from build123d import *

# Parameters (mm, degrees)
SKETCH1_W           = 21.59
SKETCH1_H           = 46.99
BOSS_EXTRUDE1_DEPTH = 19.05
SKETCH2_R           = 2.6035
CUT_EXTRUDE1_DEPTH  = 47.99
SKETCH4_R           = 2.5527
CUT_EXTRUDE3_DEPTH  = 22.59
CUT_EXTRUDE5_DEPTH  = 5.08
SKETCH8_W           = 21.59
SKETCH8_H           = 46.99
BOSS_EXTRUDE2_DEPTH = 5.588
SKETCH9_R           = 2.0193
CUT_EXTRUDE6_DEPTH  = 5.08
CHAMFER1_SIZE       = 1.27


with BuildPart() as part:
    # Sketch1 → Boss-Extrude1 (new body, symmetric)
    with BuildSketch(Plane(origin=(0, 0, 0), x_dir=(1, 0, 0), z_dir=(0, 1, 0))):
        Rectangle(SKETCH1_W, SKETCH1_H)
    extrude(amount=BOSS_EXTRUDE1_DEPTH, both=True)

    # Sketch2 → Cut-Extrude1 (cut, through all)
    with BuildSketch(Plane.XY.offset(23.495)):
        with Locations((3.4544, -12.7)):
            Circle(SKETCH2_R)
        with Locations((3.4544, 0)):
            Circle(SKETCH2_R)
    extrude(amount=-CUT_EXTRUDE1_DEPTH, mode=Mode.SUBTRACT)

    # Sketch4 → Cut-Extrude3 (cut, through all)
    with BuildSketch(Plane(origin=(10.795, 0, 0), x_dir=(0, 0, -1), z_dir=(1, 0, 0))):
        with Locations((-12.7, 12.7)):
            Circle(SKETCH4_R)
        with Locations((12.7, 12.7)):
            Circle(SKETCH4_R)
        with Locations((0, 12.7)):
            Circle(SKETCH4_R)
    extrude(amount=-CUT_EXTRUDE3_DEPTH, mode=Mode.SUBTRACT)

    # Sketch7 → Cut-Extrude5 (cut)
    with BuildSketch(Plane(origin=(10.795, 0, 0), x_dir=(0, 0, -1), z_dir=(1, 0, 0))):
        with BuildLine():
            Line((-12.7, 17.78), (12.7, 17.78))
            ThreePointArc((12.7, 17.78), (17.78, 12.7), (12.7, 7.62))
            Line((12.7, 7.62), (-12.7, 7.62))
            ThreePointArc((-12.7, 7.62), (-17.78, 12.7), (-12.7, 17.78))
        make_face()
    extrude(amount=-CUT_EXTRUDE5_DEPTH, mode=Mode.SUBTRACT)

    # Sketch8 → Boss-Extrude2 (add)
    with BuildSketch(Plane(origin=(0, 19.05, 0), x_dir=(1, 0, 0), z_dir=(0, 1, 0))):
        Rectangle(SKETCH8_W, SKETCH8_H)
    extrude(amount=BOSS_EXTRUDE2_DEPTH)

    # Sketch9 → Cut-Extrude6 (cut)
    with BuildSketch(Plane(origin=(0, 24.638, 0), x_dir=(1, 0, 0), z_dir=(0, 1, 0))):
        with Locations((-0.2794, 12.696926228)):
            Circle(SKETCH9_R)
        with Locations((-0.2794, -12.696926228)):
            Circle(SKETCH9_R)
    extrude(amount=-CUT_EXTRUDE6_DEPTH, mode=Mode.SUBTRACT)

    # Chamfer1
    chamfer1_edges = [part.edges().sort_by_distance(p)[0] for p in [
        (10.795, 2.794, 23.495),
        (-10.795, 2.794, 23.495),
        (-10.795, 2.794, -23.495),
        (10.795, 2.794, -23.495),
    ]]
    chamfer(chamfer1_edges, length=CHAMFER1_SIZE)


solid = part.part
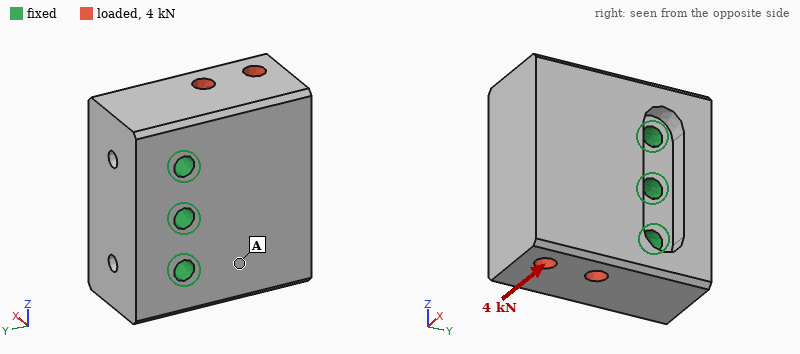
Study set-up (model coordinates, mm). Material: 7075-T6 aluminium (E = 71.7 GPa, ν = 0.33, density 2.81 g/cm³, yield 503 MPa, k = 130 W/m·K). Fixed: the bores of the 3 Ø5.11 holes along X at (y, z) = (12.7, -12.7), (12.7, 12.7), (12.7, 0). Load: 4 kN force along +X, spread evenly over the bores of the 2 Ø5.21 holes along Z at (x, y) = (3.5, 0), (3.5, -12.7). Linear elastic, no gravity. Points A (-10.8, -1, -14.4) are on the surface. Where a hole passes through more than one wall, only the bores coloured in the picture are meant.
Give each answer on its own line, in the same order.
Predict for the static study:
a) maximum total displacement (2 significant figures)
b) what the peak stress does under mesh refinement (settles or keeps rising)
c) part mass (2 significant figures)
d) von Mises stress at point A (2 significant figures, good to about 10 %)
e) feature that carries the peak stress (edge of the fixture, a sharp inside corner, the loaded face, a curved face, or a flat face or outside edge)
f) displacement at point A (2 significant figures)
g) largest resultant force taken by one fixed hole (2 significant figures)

19 µm
keeps rising
110 g
8.7 MPa
edge of the fixture
7.8 µm
1.4 kN
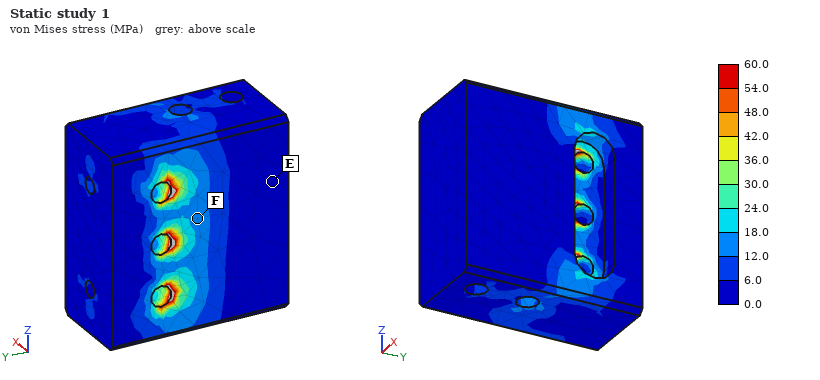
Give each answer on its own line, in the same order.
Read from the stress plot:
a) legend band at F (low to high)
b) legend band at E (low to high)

12.0 to 18.0 MPa
0.0 to 6.0 MPa
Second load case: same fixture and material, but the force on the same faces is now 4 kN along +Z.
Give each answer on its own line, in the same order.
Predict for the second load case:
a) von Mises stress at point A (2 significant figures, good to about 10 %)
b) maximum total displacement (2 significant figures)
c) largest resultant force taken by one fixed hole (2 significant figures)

4.0 MPa
9.5 µm
2.9 kN
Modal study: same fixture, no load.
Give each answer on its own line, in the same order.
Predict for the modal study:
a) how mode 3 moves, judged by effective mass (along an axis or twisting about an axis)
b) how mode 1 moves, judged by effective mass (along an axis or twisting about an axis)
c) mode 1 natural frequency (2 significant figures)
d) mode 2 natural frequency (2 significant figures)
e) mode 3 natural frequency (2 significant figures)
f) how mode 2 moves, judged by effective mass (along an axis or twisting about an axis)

twisting about Y
along X
11 kHz
15 kHz
17 kHz
along Z
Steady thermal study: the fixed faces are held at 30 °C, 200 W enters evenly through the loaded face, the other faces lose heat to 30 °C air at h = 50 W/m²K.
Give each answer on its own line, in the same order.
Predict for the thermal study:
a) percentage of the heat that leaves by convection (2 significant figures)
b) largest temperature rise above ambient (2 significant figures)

3.4 %
38 K
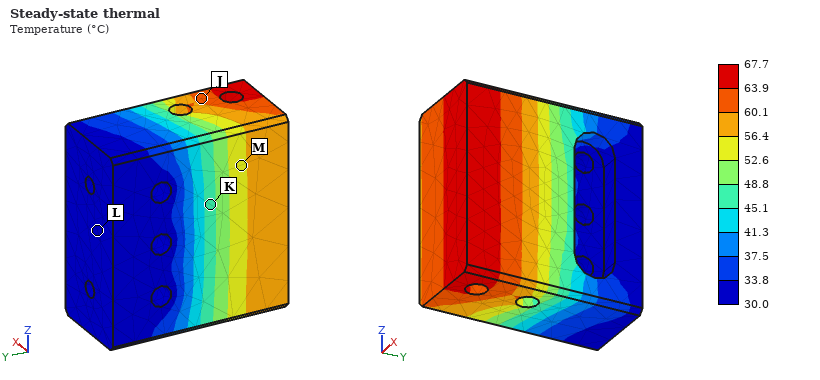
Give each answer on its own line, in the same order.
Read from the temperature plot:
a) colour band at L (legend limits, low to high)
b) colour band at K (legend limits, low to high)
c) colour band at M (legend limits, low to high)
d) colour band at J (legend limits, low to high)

30.0 to 33.8 °C
45.1 to 48.8 °C
52.6 to 56.4 °C
60.1 to 63.9 °C
